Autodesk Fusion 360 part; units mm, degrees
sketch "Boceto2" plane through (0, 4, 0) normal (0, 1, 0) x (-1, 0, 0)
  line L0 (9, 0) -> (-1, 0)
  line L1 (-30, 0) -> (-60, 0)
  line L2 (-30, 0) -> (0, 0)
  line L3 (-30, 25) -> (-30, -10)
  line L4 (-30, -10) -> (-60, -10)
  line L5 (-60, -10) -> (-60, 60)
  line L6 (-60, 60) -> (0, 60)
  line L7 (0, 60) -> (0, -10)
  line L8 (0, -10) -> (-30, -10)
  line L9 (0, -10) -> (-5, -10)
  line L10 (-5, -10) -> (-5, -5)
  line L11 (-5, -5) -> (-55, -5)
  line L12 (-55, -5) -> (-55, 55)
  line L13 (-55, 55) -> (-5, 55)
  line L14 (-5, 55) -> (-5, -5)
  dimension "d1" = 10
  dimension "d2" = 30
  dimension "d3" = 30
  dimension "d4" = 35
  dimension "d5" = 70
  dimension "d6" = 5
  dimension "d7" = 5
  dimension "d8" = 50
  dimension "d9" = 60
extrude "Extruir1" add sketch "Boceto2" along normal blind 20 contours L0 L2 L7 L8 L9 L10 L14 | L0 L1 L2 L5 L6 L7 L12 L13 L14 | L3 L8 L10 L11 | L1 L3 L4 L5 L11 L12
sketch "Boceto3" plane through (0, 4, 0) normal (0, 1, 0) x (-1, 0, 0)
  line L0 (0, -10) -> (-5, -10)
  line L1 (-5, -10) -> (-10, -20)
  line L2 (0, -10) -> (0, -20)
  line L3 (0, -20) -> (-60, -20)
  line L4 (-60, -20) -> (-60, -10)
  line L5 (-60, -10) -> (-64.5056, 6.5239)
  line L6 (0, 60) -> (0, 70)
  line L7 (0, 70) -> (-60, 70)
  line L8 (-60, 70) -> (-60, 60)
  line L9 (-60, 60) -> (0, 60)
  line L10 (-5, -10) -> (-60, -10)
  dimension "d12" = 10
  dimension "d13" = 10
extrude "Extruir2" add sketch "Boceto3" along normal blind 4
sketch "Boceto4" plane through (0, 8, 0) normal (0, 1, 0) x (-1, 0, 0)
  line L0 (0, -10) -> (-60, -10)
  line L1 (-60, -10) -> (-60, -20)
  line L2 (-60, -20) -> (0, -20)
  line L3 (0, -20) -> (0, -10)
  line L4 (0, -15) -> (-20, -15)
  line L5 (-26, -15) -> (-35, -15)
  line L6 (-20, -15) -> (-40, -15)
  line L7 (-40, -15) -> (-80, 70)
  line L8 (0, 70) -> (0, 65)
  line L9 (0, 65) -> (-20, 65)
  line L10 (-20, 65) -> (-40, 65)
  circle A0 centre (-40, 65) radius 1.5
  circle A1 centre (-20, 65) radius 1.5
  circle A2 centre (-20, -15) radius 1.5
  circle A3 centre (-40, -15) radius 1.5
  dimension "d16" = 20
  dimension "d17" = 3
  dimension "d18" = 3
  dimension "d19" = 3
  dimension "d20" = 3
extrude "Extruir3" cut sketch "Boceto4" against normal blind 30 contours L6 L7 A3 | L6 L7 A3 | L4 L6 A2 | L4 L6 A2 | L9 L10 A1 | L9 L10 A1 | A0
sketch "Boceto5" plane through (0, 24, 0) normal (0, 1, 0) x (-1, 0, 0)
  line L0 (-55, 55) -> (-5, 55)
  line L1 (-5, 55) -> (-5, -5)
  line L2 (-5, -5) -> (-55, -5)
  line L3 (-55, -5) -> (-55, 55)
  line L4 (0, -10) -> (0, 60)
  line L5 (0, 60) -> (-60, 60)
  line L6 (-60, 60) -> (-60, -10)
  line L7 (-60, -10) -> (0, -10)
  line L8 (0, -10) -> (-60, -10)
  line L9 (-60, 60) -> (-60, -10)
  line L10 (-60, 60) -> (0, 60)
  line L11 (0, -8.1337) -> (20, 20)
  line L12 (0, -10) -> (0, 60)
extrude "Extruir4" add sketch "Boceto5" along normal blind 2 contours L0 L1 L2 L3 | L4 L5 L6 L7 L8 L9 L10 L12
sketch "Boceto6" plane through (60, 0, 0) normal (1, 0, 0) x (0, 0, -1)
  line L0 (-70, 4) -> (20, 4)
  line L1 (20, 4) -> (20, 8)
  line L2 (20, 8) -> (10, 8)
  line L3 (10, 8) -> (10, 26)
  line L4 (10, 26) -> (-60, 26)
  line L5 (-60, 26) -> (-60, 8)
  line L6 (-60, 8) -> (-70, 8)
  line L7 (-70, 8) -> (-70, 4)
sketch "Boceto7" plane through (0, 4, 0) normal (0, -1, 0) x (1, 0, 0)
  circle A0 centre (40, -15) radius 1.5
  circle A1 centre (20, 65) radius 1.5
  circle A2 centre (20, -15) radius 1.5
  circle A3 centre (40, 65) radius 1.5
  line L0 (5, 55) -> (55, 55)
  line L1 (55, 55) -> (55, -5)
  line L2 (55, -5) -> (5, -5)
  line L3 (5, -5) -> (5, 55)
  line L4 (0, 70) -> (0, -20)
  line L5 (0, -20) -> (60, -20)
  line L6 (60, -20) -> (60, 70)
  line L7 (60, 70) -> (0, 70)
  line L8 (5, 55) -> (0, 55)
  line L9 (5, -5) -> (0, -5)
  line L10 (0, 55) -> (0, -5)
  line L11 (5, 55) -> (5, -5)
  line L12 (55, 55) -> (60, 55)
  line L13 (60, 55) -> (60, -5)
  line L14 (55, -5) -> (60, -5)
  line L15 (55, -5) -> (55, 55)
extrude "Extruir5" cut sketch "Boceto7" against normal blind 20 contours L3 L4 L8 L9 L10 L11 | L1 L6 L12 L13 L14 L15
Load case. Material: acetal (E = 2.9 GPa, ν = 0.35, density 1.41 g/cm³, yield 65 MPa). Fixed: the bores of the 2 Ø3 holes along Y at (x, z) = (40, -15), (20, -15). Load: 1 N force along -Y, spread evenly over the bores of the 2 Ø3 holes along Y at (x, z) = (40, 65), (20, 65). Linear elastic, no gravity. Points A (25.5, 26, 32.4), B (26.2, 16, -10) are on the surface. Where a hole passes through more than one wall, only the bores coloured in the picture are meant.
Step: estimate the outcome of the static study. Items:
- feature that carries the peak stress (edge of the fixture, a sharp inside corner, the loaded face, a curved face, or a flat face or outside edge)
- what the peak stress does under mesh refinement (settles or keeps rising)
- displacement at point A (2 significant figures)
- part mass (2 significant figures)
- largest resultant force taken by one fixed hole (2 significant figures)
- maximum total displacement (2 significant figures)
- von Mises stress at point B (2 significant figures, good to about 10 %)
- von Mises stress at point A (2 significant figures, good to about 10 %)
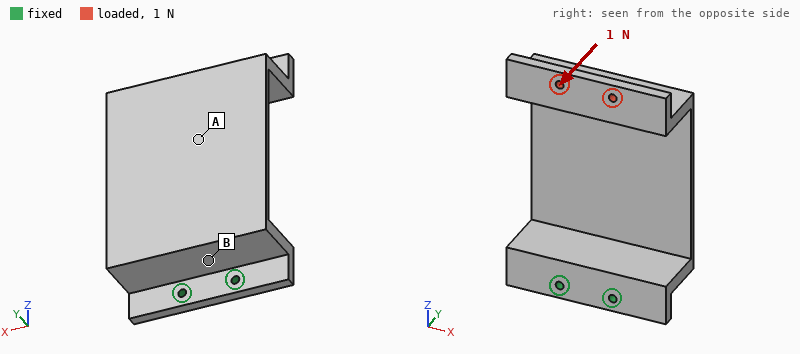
edge of the fixture
keeps rising
0.40 mm
35 g
0.58 N
1.2 mm
0.27 MPa
0.71 MPa
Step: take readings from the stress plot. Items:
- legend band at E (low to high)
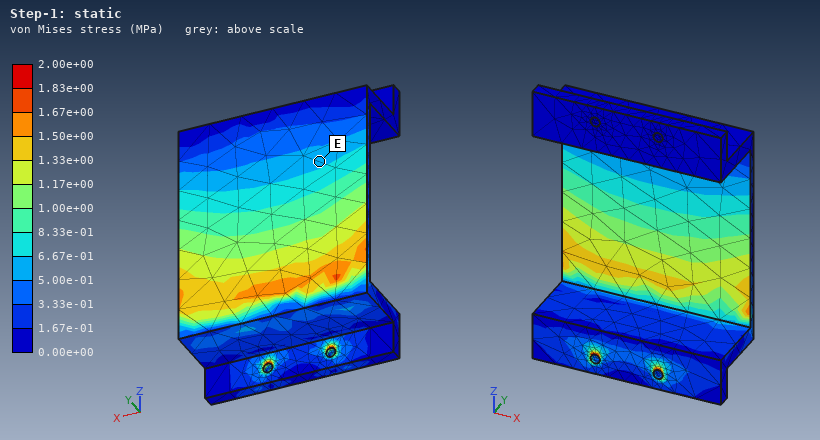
5.00e-01 to 6.67e-01 MPa
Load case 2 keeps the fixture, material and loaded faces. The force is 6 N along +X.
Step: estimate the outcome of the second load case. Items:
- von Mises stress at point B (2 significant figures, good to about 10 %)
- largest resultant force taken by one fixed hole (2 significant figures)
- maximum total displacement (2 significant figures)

1.5 MPa
21 N
1.1 mm
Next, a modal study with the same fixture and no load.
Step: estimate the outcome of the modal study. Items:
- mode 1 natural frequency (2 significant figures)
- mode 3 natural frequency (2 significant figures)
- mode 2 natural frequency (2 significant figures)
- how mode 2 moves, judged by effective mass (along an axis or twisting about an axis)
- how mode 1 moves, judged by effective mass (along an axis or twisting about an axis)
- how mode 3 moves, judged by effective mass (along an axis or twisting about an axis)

44 Hz
230 Hz
120 Hz
along X
along Y
along Z
